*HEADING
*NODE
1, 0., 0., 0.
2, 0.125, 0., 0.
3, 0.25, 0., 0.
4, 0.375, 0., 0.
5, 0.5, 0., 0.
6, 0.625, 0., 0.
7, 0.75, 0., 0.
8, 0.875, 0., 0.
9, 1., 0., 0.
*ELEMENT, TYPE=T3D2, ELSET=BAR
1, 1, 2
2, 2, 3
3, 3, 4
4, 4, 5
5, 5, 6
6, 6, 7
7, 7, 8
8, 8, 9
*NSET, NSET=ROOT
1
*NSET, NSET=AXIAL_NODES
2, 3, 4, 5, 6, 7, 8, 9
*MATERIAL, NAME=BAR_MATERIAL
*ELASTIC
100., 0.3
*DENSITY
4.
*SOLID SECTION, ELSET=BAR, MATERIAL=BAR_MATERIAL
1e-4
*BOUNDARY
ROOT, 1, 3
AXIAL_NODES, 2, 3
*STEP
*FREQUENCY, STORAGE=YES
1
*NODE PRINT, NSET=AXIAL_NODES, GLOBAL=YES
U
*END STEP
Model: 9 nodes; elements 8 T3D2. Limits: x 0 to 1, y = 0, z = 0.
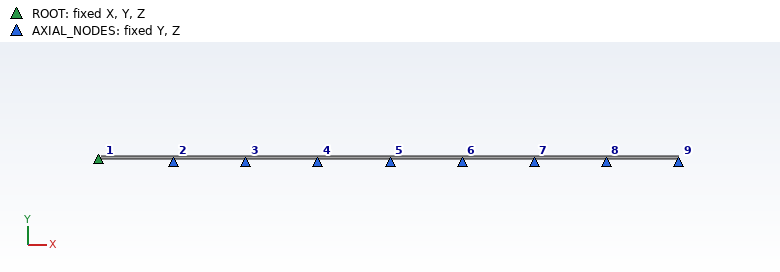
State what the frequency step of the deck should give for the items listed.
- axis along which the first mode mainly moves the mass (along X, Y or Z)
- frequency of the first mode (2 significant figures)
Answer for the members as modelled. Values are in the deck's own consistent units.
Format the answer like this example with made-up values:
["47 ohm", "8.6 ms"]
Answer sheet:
["along X", "1.3 cycles per unit time"]
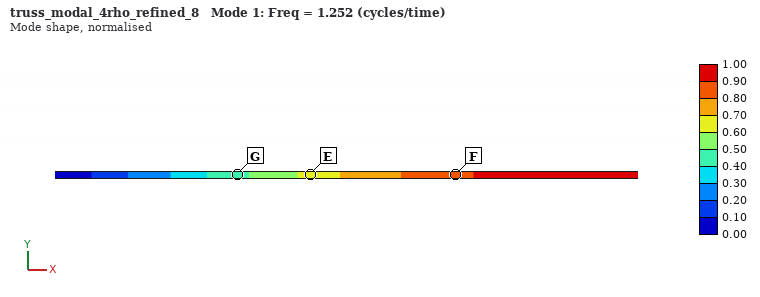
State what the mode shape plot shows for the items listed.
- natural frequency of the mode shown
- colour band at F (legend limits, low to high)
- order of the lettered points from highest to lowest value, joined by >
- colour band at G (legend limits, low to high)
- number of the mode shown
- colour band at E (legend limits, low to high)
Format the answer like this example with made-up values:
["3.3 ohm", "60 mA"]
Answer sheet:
["1.252", "0.80 to 0.90", "F > E > G", "0.40 to 0.50", "1", "0.60 to 0.70"]
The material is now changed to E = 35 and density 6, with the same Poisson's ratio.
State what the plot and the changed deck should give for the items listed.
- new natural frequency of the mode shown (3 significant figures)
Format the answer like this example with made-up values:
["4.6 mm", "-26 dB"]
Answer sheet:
["0.605"]
